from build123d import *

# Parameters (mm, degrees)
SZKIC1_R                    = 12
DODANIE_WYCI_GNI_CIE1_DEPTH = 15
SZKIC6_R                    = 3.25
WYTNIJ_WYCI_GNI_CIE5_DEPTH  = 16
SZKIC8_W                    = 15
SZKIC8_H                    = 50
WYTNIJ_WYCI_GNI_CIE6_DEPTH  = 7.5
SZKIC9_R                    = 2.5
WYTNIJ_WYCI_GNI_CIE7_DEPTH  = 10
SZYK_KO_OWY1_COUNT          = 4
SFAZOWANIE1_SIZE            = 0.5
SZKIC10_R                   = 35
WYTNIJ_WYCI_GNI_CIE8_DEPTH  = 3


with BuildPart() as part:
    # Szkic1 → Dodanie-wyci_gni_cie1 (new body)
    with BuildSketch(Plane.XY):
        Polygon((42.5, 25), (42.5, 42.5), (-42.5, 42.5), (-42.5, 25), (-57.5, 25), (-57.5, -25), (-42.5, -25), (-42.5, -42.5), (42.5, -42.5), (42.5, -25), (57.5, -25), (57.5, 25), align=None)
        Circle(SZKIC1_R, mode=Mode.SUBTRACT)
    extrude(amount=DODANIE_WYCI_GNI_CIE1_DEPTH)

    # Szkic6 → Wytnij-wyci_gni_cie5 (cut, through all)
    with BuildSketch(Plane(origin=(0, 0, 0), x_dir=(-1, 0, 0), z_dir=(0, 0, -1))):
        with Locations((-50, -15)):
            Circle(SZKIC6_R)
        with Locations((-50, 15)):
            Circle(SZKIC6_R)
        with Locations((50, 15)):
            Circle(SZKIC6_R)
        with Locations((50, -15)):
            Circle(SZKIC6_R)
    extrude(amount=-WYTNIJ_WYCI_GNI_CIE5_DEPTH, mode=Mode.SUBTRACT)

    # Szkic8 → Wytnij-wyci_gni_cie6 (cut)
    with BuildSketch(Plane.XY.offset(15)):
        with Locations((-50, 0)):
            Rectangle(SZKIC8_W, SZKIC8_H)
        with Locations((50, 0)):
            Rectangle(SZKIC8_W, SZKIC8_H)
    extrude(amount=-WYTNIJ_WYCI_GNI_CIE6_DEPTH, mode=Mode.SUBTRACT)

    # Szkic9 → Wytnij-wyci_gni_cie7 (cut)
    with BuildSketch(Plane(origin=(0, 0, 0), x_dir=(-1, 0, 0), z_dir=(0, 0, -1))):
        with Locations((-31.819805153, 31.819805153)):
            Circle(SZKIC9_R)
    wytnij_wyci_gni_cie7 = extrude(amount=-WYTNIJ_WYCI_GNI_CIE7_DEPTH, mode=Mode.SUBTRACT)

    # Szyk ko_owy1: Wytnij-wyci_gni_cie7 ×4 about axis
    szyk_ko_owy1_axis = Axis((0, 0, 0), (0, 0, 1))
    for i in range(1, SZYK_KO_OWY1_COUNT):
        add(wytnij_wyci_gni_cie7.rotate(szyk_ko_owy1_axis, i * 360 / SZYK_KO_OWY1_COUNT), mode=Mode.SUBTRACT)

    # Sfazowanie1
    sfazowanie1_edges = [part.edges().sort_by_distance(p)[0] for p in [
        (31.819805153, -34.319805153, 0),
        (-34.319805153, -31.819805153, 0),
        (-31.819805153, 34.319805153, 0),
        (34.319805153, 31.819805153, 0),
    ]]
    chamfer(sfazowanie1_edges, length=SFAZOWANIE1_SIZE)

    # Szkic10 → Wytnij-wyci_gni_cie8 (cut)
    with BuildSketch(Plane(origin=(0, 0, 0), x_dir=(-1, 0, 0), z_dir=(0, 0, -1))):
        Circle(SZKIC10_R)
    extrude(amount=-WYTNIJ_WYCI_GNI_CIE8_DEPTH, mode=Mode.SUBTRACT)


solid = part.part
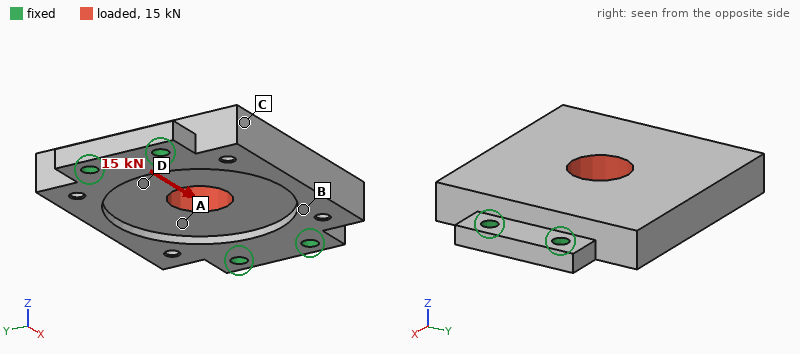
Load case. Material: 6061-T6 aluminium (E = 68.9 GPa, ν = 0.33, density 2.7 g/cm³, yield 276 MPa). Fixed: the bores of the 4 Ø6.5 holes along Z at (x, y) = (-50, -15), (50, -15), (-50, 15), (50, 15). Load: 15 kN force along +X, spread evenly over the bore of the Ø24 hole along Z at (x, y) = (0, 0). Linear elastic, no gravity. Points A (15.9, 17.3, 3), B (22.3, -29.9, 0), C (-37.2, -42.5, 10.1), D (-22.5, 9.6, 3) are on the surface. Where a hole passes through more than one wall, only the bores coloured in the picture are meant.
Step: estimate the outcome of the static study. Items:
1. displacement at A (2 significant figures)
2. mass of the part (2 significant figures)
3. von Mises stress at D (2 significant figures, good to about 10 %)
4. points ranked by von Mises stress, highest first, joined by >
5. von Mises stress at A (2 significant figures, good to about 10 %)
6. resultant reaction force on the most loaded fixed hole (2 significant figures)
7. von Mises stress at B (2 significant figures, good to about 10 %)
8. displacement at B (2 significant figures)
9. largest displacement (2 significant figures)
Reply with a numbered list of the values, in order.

1. 10 µm
2. 270 g
3. 21 MPa
4. D > A > B > C
5. 15 MPa
6. 3.8 kN
7. 7.8 MPa
8. 8.0 µm
9. 14 µm
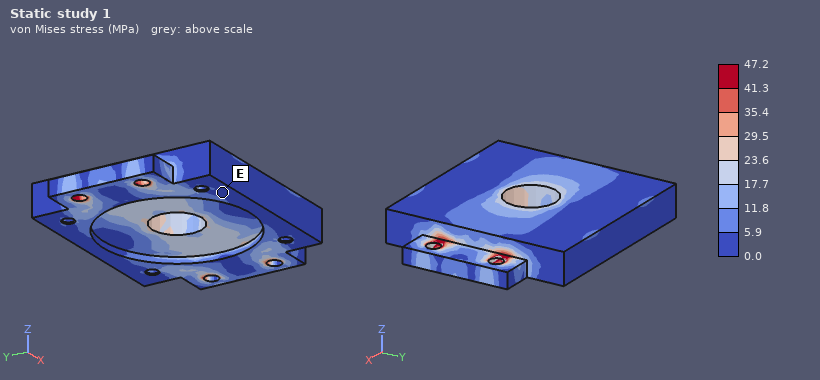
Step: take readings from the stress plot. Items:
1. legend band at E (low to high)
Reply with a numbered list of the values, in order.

1. 0.0 to 5.9 MPa
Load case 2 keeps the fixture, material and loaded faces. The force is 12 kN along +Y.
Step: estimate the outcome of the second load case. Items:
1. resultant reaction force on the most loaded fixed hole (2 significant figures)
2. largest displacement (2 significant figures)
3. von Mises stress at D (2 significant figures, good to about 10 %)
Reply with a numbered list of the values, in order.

1. 3.5 kN
2. 30 µm
3. 11 MPa
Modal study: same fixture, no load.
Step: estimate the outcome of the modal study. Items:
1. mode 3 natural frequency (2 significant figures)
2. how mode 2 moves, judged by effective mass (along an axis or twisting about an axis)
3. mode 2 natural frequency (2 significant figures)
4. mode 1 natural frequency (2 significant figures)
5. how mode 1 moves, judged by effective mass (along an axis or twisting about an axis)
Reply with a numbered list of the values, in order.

1. 8700 Hz
2. along Z
3. 4200 Hz
4. 3900 Hz
5. twisting about X
